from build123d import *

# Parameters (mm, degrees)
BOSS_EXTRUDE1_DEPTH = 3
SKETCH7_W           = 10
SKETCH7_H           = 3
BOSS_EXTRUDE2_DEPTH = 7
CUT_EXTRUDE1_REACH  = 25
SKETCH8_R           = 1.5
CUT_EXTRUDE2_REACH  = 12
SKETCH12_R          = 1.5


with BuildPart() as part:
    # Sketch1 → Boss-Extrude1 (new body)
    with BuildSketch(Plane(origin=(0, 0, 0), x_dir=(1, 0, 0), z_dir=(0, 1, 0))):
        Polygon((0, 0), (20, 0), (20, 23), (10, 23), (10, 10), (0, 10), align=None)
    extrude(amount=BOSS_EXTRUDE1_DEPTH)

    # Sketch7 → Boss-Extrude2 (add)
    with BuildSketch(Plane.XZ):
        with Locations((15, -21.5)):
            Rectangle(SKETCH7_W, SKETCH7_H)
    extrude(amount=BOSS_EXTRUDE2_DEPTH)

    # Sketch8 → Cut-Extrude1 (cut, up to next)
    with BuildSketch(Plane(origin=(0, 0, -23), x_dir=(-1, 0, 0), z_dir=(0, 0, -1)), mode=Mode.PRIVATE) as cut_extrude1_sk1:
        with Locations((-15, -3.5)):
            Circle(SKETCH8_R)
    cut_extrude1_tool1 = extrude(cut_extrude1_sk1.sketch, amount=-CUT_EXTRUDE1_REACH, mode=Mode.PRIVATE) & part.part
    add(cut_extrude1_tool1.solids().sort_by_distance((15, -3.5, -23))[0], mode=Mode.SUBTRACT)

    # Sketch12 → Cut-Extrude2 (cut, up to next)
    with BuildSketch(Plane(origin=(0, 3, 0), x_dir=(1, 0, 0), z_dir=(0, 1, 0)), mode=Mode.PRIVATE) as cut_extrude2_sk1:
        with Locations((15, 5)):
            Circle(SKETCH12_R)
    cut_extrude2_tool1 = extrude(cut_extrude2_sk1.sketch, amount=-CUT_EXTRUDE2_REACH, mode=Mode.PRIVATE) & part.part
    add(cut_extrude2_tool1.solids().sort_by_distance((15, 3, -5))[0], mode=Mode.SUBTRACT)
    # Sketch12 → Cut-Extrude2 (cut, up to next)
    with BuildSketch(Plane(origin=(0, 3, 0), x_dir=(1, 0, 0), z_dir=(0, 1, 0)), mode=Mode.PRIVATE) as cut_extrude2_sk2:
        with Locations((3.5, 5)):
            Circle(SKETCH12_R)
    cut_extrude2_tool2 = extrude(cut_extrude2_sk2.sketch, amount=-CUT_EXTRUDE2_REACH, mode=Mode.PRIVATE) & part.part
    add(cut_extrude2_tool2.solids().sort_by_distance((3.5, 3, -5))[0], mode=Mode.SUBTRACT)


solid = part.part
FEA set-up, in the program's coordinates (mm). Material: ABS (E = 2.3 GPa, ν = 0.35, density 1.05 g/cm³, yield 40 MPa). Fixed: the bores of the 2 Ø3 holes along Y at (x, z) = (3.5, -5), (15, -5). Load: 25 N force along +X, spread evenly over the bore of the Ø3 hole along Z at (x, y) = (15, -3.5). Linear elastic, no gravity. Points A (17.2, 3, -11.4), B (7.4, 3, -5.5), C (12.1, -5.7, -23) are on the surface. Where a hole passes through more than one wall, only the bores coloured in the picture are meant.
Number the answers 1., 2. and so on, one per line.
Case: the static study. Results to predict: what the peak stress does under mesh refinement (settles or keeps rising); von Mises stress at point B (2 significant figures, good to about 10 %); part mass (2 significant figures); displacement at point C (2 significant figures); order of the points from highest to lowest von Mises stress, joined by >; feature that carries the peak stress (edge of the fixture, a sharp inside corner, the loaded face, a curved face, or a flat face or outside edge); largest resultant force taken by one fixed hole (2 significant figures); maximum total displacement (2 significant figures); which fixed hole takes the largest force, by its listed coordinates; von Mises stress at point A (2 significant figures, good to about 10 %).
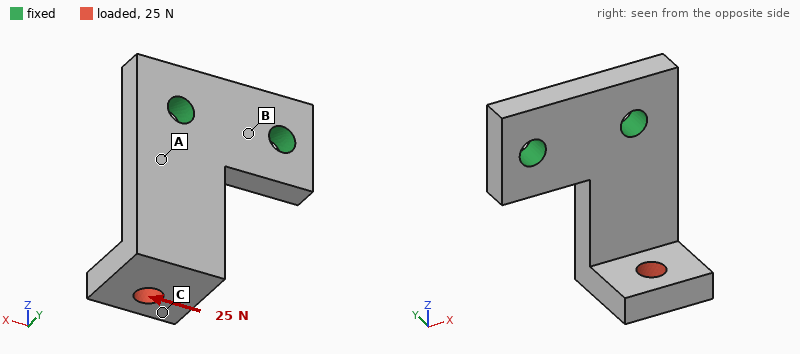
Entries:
1. keeps rising
2. 3.3 MPa
3. 1.2 g
4. 0.28 mm
5. A > B > C
6. edge of the fixture
7. 33 N
8. 0.33 mm
9. (3.5, -5)
10. 6.6 MPa
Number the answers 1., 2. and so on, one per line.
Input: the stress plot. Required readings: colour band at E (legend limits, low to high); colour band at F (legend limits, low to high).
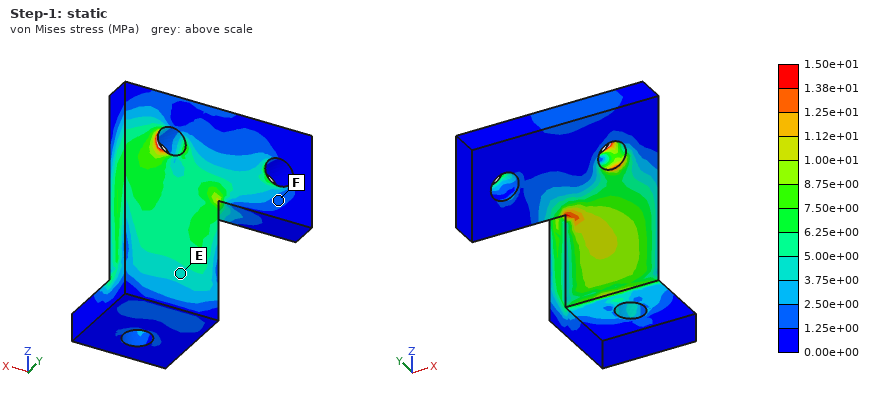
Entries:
1. 3.75e+00 to 5.00e+00 MPa
2. 1.25e+00 to 2.50e+00 MPa
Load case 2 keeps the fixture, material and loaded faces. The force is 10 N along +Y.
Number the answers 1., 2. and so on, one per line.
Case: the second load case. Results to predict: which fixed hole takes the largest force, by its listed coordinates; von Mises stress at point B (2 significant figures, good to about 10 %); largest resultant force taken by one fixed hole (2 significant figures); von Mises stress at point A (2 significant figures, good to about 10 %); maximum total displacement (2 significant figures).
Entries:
1. (15, -5)
2. 1.8 MPa
3. 11 N
4. 6.1 MPa
5. 0.34 mm
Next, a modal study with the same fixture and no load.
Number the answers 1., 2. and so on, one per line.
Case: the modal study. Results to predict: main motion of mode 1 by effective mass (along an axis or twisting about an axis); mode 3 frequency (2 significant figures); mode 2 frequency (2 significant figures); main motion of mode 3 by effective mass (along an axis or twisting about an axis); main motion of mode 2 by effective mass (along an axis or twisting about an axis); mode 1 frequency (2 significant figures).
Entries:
1. along Y
2. 5600 Hz
3. 3200 Hz
4. along X
5. along X
6. 1600 Hz
